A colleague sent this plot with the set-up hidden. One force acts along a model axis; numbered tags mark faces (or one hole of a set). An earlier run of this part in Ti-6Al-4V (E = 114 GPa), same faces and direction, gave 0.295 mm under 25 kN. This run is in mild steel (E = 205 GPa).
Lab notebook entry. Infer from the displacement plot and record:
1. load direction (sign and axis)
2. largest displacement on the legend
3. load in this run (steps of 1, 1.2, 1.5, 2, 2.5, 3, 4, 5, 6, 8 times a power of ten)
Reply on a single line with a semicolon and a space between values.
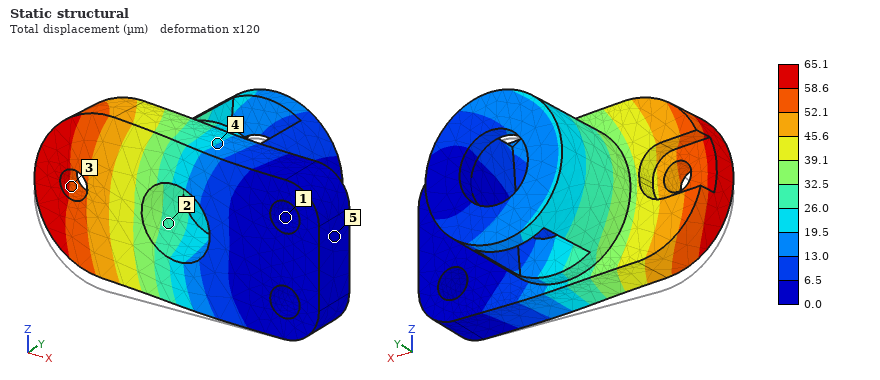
+Z; 65.1 µm; 10 kN
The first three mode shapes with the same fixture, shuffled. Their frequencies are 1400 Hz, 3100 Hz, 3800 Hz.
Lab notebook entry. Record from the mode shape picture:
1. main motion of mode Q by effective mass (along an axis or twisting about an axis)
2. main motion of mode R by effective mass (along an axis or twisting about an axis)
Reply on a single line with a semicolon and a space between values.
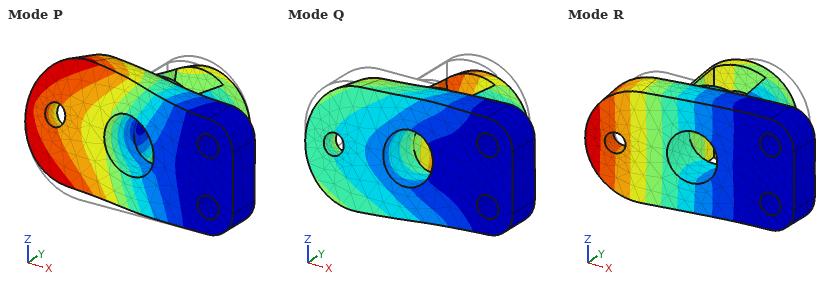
along Z; along Y
